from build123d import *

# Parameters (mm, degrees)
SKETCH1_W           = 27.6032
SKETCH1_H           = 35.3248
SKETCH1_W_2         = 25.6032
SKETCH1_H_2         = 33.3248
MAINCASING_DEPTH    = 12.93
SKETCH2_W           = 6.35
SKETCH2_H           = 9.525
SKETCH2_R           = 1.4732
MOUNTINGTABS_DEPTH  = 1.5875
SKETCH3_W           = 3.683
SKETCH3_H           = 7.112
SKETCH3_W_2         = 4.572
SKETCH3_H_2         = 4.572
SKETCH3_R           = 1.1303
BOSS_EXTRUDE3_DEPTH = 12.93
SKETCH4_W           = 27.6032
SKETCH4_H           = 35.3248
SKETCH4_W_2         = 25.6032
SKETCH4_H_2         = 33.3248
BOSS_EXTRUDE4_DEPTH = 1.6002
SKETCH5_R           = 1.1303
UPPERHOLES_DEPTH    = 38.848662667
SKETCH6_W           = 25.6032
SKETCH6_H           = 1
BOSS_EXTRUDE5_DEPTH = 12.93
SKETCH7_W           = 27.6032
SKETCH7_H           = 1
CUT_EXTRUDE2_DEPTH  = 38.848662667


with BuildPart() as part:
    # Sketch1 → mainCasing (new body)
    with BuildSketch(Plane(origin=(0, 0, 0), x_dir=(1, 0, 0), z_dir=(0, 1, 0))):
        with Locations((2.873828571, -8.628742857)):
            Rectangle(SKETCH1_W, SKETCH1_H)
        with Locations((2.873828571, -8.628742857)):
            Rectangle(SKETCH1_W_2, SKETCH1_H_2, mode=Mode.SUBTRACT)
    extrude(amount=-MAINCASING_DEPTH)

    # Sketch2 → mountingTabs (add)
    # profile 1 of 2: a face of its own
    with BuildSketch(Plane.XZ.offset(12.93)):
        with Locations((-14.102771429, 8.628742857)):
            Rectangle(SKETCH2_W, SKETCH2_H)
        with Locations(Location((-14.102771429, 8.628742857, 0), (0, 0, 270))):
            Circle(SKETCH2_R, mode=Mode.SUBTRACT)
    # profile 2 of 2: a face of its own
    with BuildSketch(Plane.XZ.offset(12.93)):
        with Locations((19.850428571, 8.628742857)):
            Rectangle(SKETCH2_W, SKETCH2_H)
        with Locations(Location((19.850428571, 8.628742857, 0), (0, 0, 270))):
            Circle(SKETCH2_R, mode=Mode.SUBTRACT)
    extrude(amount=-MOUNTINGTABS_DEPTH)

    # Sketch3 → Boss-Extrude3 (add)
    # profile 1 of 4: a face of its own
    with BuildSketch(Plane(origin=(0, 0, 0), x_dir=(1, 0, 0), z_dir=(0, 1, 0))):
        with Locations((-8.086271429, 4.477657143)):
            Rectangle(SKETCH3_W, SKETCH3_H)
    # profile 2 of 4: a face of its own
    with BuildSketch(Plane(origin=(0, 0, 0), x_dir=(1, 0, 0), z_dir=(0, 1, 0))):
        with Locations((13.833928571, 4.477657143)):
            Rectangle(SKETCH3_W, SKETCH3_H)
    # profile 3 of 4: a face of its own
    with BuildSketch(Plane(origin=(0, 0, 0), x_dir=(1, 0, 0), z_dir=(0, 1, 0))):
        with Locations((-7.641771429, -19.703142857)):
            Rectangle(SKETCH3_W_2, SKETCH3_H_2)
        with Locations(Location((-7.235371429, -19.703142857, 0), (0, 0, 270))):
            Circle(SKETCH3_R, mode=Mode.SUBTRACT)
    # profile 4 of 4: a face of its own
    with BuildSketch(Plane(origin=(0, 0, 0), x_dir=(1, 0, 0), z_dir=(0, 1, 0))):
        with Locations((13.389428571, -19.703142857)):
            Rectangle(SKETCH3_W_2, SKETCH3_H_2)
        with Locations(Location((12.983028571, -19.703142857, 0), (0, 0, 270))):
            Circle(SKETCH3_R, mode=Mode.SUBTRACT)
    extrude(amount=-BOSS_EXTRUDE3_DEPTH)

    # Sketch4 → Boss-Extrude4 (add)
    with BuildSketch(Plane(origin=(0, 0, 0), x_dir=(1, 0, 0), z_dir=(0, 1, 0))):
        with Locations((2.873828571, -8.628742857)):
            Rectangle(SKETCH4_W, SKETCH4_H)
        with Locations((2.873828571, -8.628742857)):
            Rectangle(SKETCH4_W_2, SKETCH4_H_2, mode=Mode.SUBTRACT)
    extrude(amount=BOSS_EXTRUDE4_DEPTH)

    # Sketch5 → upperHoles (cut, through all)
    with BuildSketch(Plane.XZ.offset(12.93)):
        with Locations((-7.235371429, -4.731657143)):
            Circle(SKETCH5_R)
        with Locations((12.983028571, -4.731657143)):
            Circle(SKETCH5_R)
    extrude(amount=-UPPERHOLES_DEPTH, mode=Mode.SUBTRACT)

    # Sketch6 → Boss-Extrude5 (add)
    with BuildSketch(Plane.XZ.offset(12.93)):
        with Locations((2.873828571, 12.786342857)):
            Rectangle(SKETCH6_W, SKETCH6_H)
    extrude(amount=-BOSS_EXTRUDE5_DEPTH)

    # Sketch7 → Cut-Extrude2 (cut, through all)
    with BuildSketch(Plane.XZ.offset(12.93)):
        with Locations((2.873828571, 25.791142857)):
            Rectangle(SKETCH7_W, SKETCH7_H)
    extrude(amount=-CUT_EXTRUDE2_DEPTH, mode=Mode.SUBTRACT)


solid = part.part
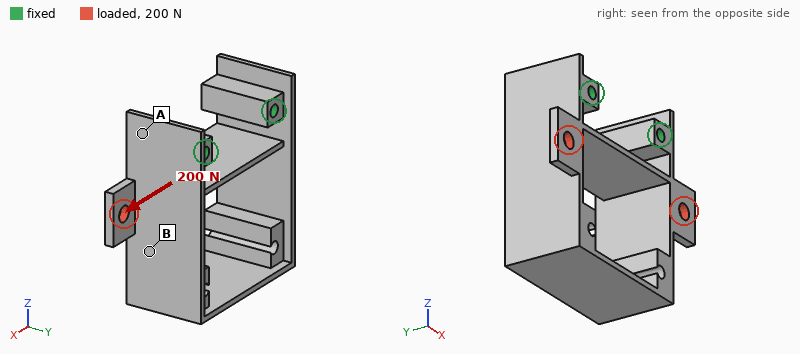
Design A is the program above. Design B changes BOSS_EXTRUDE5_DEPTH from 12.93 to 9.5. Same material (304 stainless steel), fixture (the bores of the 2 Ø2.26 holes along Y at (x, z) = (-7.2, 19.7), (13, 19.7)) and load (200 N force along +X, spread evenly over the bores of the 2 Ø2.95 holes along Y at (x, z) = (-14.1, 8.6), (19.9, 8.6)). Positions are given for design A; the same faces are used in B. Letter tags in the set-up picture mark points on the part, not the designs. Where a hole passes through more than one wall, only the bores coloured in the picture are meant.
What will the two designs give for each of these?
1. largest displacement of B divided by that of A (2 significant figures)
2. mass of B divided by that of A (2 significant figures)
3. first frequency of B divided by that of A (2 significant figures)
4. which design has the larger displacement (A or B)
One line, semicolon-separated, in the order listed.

1.1; 0.97; 0.97; B
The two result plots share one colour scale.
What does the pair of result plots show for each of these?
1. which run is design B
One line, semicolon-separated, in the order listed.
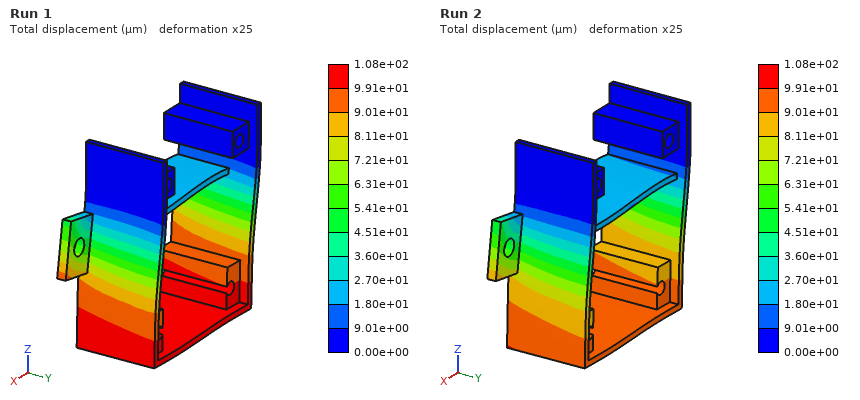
Run 1
